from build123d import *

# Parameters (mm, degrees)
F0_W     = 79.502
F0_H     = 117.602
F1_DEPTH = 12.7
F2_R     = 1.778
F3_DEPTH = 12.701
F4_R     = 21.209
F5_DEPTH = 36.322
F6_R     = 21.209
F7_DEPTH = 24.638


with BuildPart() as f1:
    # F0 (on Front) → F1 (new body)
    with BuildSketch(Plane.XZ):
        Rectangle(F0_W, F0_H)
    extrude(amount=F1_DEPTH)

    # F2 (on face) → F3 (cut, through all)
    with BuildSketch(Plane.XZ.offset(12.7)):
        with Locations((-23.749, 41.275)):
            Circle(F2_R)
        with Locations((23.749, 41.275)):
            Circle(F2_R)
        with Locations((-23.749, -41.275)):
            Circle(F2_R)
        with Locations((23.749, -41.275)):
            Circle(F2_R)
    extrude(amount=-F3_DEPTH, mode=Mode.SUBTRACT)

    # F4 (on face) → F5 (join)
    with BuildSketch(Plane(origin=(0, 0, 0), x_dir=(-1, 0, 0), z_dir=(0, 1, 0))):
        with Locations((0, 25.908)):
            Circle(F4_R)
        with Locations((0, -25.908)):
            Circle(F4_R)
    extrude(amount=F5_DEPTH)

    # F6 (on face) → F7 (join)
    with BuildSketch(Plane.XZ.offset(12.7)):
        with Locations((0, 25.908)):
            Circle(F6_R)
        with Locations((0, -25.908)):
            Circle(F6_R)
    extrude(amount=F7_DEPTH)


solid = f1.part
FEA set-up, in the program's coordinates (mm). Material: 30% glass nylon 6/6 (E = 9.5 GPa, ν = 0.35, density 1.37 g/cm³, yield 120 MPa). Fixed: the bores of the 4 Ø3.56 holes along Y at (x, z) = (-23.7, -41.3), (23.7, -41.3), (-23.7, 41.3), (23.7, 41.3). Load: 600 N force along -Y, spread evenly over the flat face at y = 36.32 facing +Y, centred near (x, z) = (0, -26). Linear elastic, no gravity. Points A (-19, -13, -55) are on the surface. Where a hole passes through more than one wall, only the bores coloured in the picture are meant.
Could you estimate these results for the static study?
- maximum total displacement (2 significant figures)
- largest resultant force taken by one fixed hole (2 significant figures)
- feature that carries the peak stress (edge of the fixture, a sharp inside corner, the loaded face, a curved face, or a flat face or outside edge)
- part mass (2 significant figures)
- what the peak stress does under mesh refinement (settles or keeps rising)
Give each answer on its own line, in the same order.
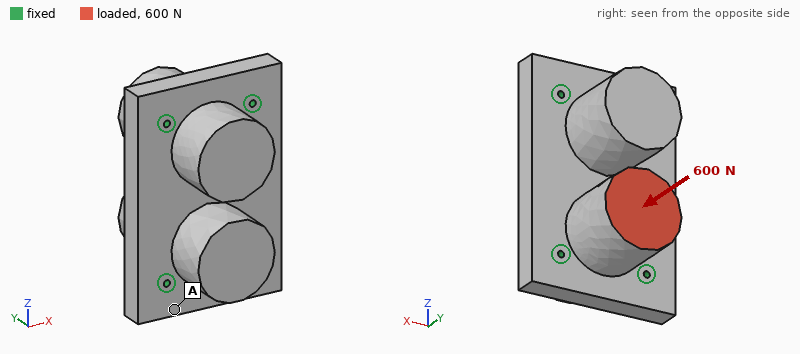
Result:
16 µm
250 N
edge of the fixture
400 g
keeps rising
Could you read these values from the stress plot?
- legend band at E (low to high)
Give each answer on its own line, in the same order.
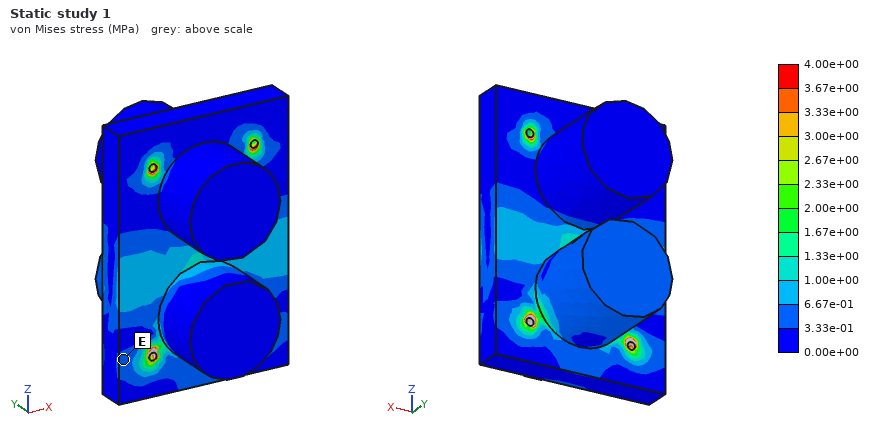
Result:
3.33e-01 to 6.67e-01 MPa
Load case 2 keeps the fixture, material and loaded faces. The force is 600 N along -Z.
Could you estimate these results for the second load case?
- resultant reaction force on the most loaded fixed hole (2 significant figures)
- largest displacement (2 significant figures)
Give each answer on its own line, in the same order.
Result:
250 N
59 µm
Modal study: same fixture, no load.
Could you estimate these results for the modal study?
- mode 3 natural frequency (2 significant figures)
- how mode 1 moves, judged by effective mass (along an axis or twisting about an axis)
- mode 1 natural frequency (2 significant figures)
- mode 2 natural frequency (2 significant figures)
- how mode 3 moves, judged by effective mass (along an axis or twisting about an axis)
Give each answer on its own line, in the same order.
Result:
4200 Hz
along Y
1800 Hz
3400 Hz
along Z
